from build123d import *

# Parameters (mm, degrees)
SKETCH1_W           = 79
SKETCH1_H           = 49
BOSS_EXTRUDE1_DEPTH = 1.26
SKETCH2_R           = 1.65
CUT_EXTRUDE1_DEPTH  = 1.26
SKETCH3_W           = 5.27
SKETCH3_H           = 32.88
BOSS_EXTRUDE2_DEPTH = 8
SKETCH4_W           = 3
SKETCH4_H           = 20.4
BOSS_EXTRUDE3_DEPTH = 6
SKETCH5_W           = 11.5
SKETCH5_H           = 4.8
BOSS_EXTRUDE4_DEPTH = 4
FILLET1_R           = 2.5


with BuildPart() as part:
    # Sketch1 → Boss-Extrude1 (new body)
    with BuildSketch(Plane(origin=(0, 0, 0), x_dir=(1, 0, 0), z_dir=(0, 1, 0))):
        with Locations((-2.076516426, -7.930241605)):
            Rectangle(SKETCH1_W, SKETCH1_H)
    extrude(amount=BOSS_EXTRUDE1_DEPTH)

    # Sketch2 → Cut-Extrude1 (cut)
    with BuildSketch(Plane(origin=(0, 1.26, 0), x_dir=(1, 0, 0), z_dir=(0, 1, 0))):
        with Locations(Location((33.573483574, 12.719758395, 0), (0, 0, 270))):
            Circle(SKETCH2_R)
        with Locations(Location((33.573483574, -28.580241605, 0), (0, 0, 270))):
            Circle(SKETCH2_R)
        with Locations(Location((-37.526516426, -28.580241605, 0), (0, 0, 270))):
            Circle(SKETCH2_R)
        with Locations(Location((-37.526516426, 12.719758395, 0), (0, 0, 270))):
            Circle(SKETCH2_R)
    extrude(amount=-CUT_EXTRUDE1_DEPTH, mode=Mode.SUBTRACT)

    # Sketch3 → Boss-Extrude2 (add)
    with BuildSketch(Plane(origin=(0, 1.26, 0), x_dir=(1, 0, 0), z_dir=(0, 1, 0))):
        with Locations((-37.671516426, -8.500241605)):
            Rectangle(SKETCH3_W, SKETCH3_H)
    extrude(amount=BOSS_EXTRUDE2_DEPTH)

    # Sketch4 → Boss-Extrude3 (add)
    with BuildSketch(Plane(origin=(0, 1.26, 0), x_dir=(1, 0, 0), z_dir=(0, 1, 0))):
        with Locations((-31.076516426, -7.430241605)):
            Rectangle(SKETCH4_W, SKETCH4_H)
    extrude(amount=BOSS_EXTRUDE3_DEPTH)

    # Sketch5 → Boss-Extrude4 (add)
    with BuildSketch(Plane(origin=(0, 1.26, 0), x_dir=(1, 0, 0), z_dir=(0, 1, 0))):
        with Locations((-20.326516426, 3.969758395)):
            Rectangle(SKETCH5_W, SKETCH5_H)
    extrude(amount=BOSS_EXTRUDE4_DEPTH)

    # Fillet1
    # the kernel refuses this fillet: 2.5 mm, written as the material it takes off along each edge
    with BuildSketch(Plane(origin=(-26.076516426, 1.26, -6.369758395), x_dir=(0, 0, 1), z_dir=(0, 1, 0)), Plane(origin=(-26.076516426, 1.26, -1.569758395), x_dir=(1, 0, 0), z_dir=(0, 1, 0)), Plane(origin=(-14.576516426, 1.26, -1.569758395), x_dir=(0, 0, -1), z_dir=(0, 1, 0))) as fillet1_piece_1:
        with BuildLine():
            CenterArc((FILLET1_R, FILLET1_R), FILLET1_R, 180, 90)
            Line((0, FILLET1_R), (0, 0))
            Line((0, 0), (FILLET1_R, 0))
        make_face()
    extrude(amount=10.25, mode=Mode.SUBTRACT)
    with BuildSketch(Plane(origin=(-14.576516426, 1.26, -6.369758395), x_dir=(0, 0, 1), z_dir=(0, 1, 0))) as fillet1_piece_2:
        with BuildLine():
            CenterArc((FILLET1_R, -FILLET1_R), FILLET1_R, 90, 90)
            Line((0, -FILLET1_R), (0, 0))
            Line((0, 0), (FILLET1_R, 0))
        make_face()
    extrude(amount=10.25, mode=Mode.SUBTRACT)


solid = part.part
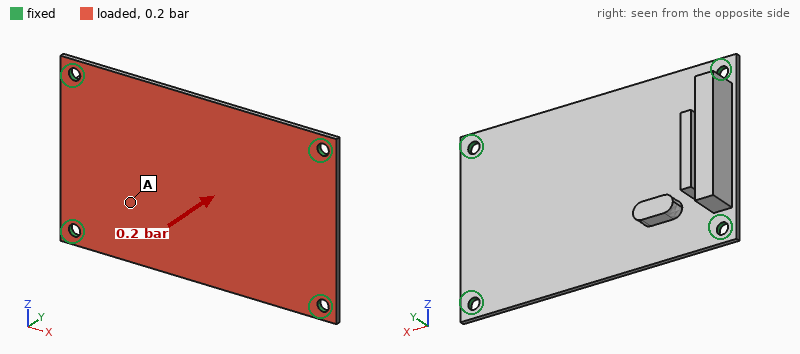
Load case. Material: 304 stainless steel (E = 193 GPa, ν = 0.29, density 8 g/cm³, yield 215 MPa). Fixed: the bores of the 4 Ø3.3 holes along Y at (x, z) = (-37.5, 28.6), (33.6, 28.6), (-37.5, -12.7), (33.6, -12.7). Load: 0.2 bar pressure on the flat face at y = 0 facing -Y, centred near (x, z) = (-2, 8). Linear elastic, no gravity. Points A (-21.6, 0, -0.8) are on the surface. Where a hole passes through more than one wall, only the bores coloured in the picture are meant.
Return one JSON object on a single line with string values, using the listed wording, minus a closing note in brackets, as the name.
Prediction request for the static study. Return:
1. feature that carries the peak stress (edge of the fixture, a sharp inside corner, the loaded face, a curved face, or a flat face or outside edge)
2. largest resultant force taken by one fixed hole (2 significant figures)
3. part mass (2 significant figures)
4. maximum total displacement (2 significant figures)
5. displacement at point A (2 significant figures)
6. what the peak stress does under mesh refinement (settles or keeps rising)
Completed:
{"feature that carries the peak stress": "edge of the fixture", "largest resultant force taken by one fixed hole": "22 N", "part mass": "54 g", "maximum total displacement": "47 µm", "displacement at point A": "22 µm", "what the peak stress does under mesh refinement": "keeps rising"}
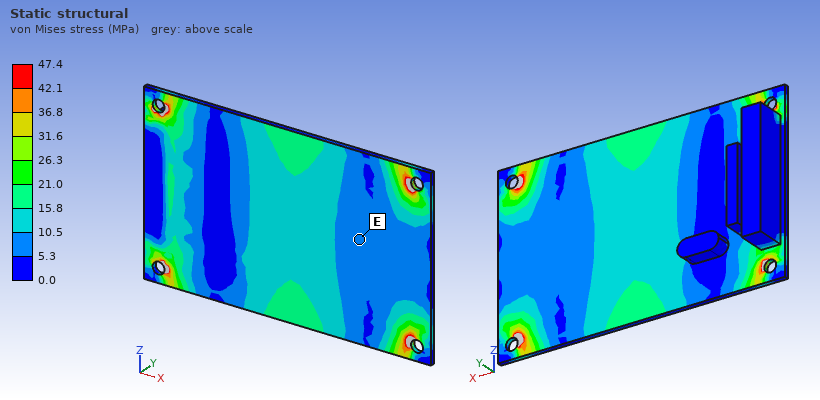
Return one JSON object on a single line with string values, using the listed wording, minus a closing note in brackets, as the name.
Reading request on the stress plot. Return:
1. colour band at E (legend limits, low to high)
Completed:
{"colour band at E": "5.3 to 10.5 MPa"}
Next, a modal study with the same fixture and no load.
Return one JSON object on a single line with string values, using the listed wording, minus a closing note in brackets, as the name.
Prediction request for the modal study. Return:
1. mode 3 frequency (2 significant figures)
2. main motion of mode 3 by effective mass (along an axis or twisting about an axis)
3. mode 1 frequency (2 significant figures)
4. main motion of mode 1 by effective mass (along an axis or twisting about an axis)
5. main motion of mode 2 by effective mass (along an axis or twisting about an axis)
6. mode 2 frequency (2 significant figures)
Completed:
{"mode 3 frequency": "3000 Hz", "main motion of mode 3 by effective mass": "twisting about Z", "mode 1 frequency": "1200 Hz", "main motion of mode 1 by effective mass": "along Y", "main motion of mode 2 by effective mass": "twisting about X", "mode 2 frequency": "1900 Hz"}
